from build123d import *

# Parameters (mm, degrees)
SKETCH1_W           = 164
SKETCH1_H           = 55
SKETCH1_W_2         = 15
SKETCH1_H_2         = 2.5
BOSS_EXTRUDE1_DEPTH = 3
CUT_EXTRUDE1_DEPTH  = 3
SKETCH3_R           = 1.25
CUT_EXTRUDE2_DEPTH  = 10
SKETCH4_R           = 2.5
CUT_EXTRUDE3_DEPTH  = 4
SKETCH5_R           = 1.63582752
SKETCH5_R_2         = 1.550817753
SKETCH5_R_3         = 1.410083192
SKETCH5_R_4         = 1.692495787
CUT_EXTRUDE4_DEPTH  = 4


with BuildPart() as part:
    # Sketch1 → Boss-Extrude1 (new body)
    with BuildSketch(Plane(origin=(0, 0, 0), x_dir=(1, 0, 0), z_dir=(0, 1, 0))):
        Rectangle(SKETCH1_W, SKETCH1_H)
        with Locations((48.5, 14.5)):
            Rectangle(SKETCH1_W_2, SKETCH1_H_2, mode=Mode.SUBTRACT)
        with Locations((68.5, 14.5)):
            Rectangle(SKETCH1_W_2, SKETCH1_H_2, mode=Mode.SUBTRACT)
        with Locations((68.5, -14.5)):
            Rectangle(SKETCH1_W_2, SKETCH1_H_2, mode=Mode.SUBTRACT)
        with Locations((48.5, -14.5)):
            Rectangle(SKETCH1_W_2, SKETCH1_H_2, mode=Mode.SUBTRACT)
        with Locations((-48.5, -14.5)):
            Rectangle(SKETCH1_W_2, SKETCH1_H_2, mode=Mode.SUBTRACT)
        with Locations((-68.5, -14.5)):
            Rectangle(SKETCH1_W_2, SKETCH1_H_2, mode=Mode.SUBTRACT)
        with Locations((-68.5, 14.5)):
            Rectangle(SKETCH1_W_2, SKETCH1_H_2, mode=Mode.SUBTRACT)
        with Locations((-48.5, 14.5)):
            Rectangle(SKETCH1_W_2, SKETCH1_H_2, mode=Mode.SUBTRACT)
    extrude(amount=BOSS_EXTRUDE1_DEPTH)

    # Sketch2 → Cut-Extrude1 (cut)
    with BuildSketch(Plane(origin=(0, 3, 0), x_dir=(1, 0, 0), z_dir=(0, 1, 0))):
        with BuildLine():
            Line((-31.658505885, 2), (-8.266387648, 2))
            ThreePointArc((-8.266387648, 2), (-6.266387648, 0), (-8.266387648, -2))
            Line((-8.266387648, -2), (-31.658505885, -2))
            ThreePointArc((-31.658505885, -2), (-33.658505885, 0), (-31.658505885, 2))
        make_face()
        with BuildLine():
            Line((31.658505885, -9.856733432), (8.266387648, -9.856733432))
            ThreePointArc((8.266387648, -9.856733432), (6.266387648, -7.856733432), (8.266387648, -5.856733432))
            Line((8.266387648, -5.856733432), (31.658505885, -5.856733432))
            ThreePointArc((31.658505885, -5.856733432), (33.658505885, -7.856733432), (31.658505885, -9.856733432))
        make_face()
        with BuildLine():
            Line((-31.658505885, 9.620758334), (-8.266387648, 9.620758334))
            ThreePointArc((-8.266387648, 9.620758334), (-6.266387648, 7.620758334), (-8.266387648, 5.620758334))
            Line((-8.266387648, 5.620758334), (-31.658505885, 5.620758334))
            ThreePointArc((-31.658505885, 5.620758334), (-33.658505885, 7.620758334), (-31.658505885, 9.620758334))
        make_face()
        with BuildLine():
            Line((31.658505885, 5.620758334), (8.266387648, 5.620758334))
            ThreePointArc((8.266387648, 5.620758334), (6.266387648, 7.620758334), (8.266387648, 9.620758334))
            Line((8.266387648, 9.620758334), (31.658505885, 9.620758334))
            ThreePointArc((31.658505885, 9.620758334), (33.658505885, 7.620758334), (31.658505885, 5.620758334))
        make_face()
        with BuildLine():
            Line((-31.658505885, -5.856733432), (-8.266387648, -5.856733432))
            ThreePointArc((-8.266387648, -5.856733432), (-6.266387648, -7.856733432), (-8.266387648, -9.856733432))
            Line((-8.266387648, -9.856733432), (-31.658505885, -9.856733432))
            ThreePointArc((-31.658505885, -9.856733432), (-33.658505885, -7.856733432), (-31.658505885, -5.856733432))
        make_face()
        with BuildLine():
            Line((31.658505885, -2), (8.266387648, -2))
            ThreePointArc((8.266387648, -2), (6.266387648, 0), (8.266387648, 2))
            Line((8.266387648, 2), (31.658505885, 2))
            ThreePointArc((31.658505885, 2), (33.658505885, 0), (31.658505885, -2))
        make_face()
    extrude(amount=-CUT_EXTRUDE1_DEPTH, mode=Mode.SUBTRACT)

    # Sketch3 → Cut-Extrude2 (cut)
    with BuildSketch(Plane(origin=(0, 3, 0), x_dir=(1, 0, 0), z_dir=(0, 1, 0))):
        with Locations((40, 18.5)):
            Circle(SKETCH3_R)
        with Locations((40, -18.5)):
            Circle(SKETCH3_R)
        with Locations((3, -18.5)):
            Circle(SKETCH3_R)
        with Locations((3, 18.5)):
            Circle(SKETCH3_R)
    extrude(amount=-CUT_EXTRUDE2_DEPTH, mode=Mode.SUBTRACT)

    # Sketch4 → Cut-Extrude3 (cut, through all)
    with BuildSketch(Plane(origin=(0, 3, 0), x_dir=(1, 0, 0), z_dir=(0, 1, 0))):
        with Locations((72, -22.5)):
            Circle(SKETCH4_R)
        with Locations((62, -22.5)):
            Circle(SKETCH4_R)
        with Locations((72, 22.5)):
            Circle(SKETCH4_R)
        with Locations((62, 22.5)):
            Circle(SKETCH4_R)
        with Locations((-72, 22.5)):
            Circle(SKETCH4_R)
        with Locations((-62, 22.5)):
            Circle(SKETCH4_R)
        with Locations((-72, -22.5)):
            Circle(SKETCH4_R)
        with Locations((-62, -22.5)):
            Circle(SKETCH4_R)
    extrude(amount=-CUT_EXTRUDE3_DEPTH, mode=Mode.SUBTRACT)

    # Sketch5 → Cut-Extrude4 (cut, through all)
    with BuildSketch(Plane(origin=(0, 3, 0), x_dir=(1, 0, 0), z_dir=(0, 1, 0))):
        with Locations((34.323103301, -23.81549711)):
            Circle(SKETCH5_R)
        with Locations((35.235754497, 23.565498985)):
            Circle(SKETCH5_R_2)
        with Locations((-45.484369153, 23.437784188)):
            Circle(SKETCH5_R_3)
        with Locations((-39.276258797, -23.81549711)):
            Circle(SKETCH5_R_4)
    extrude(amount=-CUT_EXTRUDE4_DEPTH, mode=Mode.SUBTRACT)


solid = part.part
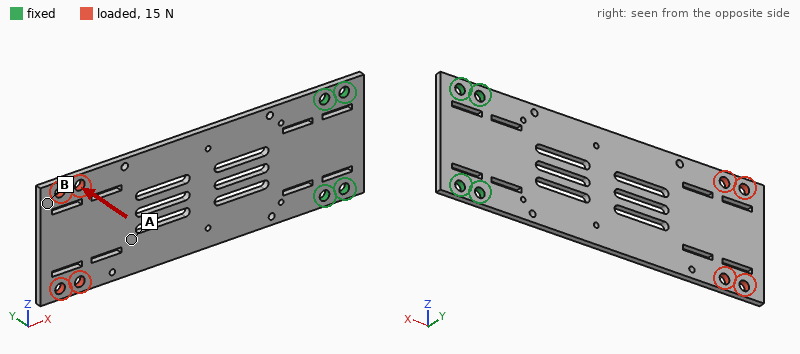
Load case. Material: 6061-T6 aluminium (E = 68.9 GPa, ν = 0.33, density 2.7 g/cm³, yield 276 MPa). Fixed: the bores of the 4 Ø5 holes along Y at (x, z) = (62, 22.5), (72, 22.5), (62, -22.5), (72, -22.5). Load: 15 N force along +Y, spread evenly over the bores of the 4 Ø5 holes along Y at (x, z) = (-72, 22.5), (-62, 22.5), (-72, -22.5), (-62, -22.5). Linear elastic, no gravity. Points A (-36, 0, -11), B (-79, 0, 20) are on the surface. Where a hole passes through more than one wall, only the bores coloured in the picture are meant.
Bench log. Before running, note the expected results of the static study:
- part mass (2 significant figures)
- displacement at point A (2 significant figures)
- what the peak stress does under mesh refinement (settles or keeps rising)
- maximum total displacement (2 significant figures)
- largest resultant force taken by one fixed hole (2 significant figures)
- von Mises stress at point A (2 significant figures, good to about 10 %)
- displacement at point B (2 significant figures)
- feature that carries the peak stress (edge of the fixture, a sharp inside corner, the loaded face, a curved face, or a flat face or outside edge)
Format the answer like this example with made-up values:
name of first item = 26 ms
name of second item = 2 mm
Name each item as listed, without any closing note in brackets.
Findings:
part mass = 64 g
displacement at point A = 0.97 mm
what the peak stress does under mesh refinement = keeps rising
maximum total displacement = 1.8 mm
largest resultant force taken by one fixed hole = 33 N
von Mises stress at point A = 6.2 MPa
displacement at point B = 1.7 mm
feature that carries the peak stress = edge of the fixture
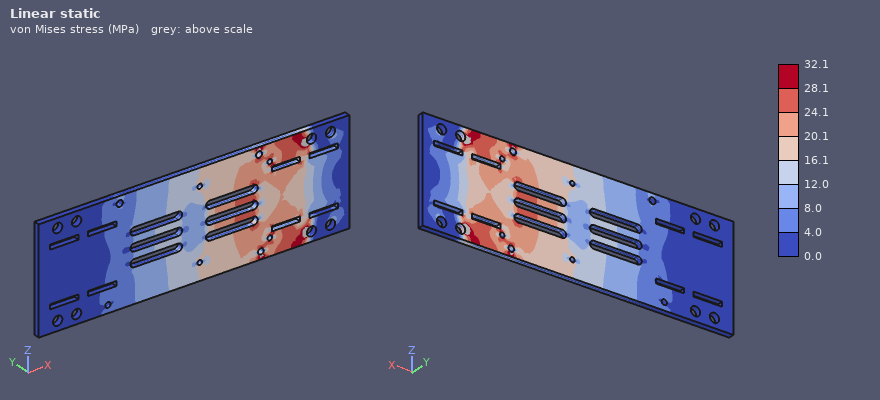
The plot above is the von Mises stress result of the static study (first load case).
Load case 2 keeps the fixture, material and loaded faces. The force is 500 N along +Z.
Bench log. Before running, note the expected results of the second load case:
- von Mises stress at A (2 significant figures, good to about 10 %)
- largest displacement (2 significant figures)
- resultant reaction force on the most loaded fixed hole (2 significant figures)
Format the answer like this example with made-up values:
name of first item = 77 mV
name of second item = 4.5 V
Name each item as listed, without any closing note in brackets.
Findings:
von Mises stress at A = 20 MPa
largest displacement = 0.23 mm
resultant reaction force on the most loaded fixed hole = 1.3 kN
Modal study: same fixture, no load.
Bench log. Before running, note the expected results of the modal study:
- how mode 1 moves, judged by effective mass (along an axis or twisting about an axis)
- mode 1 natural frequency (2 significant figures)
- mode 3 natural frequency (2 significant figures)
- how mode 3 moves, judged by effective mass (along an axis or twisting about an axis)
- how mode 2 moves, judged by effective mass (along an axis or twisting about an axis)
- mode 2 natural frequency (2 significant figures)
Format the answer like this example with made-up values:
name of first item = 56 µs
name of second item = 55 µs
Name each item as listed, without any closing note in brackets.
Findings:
how mode 1 moves, judged by effective mass = along Y
mode 1 natural frequency = 110 Hz
mode 3 natural frequency = 720 Hz
how mode 3 moves, judged by effective mass = along Y
how mode 2 moves, judged by effective mass = twisting about X
mode 2 natural frequency = 590 Hz
